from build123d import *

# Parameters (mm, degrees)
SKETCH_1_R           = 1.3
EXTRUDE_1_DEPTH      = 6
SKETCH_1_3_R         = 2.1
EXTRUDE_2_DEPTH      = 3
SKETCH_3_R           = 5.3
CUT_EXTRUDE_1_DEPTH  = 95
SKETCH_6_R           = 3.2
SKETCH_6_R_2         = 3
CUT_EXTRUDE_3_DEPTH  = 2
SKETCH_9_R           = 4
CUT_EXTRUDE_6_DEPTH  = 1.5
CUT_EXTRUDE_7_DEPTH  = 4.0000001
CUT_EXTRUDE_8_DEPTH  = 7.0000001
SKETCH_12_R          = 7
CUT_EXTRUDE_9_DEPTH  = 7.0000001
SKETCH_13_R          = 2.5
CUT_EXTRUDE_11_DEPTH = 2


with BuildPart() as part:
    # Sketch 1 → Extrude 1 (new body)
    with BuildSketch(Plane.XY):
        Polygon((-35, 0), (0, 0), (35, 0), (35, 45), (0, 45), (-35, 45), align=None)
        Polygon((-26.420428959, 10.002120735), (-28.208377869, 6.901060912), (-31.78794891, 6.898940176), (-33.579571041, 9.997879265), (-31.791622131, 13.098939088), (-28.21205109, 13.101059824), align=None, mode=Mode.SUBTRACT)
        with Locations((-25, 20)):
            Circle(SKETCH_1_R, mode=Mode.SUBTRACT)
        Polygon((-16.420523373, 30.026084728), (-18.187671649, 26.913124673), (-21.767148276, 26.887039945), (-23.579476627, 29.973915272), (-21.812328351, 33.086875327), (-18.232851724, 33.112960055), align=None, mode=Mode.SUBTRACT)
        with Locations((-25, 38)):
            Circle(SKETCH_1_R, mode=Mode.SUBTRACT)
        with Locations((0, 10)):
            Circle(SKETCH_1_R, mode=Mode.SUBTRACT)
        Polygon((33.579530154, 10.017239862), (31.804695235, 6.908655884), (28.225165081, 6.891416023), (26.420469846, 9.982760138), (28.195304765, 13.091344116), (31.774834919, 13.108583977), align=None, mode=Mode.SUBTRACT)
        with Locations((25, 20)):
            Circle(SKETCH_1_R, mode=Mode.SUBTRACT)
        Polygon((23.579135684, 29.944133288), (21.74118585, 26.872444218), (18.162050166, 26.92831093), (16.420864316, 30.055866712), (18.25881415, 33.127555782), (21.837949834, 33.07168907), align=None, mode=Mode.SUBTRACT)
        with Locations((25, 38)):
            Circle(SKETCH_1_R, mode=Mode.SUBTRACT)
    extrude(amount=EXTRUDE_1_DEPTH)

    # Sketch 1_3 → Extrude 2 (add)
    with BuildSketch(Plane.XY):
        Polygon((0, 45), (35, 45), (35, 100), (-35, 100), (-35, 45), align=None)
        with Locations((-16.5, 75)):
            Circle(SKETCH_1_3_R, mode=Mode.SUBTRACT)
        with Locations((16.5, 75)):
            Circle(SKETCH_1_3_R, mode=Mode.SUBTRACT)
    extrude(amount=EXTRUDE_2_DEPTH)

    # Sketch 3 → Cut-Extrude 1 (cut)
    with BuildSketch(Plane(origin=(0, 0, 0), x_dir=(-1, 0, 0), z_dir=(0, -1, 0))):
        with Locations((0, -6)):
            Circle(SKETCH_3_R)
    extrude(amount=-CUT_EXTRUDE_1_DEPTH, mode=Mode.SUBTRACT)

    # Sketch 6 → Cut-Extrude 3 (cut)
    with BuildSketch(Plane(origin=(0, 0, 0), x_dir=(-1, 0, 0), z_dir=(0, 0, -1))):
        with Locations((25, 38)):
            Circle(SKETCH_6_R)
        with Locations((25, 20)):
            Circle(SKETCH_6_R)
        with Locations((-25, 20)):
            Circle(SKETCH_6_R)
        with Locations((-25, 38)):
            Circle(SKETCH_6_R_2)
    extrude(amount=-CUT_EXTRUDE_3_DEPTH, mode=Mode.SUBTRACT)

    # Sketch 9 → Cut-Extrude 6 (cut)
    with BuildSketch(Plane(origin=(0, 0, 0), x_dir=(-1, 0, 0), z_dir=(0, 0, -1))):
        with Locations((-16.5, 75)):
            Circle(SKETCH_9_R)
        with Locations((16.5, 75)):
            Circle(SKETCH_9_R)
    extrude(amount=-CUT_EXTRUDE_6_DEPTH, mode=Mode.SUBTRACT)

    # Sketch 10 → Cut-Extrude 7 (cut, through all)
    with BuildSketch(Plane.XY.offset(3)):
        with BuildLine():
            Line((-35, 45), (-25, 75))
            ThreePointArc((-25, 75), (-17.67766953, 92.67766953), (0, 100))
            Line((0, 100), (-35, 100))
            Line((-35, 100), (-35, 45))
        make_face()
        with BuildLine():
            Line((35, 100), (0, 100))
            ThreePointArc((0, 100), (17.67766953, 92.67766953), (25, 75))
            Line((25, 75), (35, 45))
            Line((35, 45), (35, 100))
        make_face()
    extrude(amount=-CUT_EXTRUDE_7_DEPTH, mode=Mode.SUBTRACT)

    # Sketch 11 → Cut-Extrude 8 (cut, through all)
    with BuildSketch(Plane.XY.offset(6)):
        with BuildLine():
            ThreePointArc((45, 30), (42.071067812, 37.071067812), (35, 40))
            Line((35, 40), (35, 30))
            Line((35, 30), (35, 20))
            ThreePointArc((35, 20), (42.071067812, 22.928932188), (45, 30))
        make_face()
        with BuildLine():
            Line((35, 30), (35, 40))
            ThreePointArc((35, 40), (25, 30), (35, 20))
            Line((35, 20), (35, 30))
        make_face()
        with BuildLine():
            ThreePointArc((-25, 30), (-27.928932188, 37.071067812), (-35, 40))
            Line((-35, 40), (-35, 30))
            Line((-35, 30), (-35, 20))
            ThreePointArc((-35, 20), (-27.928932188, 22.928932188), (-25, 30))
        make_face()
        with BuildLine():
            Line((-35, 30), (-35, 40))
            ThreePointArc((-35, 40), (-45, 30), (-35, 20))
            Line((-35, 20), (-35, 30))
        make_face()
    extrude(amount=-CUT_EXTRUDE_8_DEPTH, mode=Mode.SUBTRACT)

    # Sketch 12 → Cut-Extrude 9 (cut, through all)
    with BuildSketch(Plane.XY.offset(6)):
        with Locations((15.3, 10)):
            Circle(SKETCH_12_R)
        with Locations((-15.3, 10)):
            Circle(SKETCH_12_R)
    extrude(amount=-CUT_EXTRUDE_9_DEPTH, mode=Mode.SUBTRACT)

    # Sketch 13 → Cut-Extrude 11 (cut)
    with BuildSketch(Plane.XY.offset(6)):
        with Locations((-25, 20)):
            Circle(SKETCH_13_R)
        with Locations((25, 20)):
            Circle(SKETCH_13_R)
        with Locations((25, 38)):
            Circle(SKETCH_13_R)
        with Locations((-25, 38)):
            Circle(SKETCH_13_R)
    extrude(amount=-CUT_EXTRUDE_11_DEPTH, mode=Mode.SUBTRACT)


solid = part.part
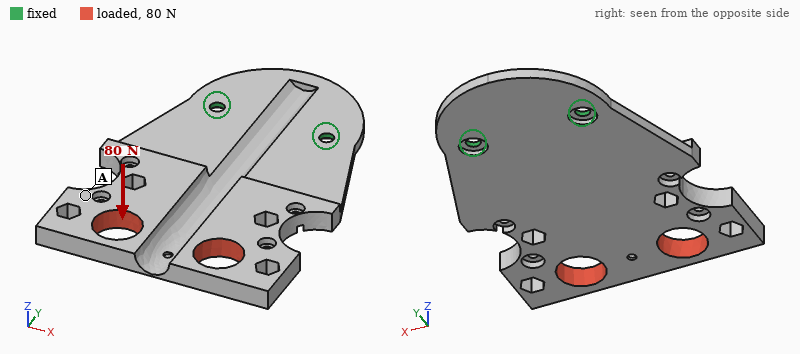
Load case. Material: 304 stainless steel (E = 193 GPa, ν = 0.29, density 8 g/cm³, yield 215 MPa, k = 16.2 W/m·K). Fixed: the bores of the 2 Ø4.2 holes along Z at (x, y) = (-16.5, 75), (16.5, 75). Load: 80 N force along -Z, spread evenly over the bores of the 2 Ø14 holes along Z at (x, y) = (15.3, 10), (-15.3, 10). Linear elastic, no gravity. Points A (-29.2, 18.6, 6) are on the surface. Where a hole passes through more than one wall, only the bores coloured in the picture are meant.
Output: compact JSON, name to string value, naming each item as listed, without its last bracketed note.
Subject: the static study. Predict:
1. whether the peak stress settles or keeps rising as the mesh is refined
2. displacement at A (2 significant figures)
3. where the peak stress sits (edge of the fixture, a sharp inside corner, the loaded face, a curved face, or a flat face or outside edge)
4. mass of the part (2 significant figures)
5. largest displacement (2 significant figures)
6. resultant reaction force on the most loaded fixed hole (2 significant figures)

{"whether the peak stress settles or keeps rising as the mesh is refined": "keeps rising", "displacement at A": "0.32 mm", "where the peak stress sits": "edge of the fixture", "mass of the part": "160 g", "largest displacement": "0.45 mm", "resultant reaction force on the most loaded fixed hole": "45 N"}
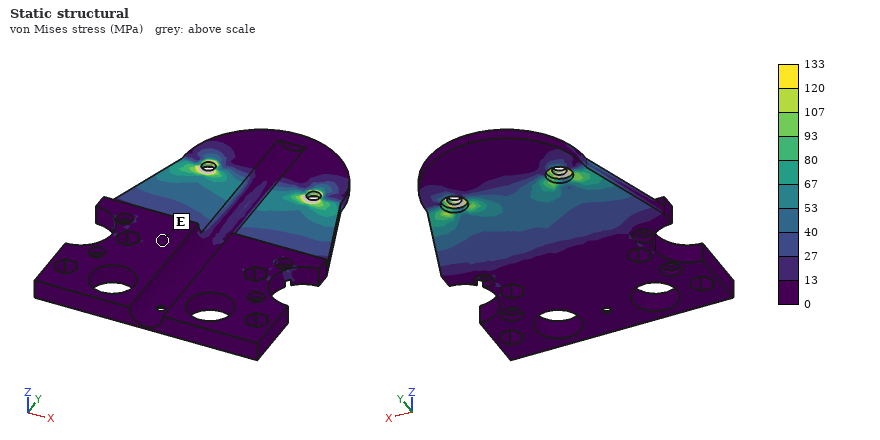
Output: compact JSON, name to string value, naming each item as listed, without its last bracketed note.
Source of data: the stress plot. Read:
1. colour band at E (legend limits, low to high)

{"colour band at E": "0 to 13 MPa"}
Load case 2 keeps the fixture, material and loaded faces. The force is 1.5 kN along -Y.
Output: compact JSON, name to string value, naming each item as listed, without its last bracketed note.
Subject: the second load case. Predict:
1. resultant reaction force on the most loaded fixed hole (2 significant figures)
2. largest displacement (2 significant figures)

{"resultant reaction force on the most loaded fixed hole": "750 N", "largest displacement": "0.19 mm"}
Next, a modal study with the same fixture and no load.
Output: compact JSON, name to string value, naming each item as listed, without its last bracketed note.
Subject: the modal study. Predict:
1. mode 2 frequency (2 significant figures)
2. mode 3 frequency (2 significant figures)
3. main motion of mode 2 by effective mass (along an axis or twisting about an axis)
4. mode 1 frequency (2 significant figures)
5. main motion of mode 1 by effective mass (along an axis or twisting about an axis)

{"mode 2 frequency": "980 Hz", "mode 3 frequency": "1900 Hz", "main motion of mode 2 by effective mass": "twisting about Y", "mode 1 frequency": "290 Hz", "main motion of mode 1 by effective mass": "along Z"}
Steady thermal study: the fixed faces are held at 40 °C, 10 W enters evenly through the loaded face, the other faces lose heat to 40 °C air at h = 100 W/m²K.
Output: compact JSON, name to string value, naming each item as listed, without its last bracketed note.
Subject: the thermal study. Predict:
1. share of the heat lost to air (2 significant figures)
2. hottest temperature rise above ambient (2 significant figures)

{"share of the heat lost to air": "99 %", "hottest temperature rise above ambient": "31 K"}
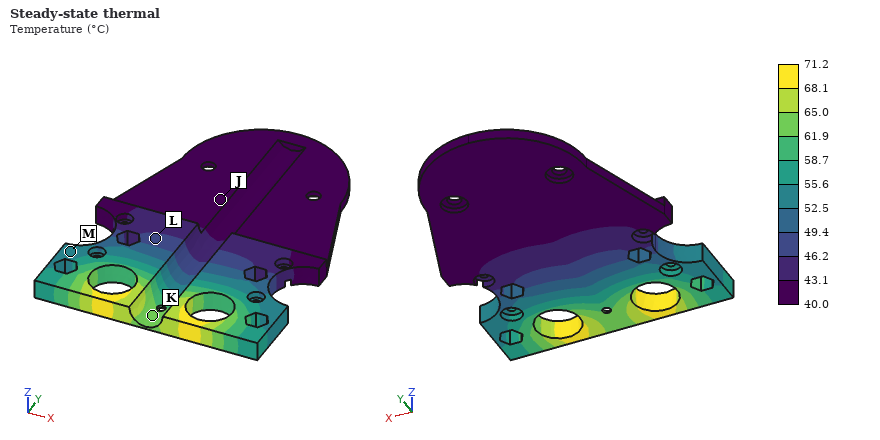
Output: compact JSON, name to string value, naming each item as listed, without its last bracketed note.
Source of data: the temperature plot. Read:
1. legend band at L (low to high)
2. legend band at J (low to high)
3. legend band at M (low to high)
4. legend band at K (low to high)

{"legend band at L": "46.2 to 49.4 °C", "legend band at J": "40.0 to 43.1 °C", "legend band at M": "52.5 to 55.6 °C", "legend band at K": "61.9 to 65.0 °C"}
